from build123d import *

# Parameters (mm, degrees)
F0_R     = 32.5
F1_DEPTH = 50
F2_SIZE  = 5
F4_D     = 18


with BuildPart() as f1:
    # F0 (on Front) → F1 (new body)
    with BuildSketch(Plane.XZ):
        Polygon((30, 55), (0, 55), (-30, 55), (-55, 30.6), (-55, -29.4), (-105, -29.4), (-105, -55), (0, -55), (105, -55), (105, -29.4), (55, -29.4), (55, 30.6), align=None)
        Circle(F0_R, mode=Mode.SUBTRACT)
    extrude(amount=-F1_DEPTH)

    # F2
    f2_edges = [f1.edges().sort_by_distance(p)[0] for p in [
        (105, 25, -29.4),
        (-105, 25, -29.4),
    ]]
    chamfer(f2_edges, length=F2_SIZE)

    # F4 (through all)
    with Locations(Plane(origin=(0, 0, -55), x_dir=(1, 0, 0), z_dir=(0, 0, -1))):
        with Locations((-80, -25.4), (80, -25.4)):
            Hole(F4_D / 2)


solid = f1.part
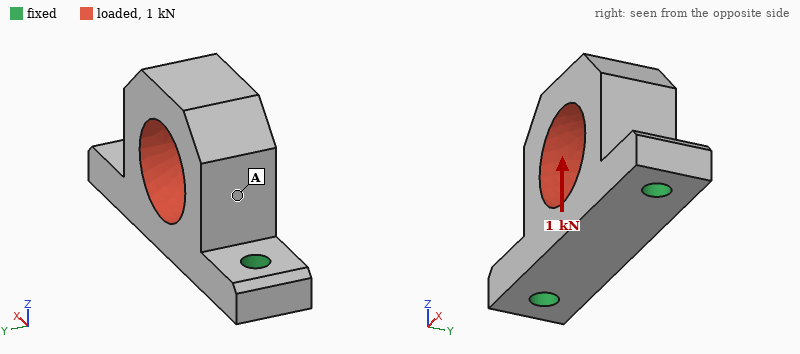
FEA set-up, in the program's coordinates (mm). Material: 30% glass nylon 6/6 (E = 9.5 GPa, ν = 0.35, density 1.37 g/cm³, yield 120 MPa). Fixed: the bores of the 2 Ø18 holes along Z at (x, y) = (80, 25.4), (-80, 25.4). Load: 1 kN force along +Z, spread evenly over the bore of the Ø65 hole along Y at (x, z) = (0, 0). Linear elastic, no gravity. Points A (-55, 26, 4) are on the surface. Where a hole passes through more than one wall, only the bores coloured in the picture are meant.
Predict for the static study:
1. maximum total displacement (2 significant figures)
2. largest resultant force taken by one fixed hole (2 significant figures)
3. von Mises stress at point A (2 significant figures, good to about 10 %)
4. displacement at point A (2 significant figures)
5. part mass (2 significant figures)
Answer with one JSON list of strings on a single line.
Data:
["13 µm", "510 N", "0.45 MPa", "9.1 µm", "720 g"]
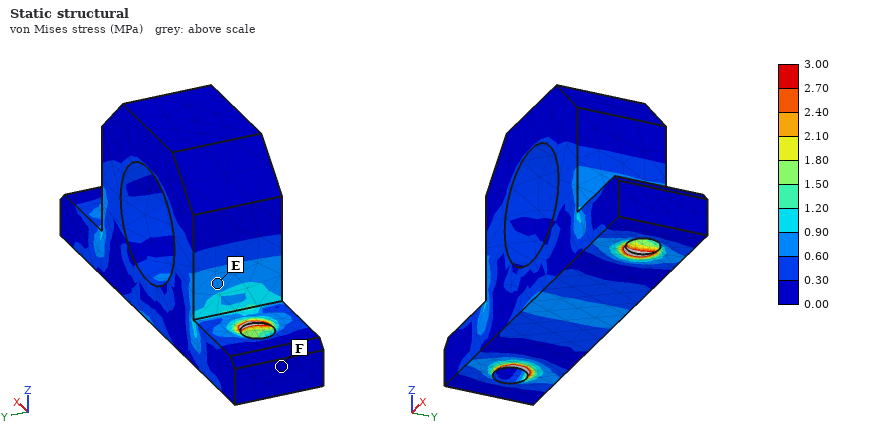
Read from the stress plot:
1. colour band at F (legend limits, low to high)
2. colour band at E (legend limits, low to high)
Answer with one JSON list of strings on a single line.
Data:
["0.00 to 0.30 MPa", "0.60 to 0.90 MPa"]
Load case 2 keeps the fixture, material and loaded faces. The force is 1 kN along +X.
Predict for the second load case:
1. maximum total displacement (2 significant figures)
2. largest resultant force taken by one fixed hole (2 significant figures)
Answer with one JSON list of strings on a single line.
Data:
["18 µm", "590 N"]
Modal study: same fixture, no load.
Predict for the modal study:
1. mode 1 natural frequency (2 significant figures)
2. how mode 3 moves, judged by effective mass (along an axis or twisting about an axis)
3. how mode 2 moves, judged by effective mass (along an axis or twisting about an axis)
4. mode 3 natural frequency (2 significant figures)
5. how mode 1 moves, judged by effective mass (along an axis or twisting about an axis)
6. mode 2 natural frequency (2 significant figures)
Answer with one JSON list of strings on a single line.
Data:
["800 Hz", "along Z", "along X", "2200 Hz", "along Y", "1800 Hz"]
